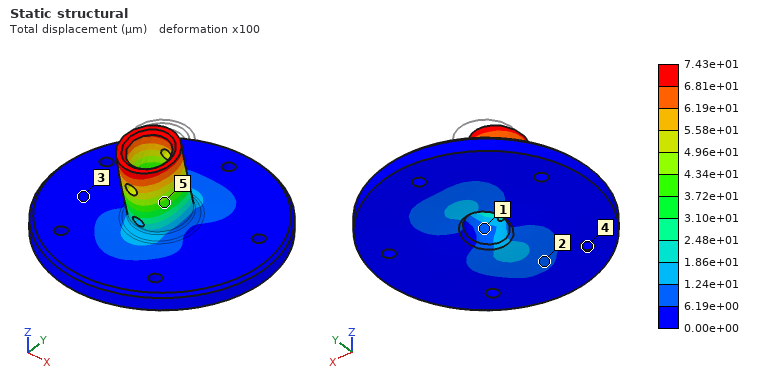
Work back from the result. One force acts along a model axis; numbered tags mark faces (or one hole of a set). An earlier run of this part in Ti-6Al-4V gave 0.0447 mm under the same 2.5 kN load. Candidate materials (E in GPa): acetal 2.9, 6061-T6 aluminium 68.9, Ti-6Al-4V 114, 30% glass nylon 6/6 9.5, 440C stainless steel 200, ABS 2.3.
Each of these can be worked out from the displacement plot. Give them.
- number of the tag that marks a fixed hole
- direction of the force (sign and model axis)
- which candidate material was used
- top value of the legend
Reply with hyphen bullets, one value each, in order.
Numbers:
- 4
- -Y
- 6061-T6 aluminium
- 7.43e+01 µm
